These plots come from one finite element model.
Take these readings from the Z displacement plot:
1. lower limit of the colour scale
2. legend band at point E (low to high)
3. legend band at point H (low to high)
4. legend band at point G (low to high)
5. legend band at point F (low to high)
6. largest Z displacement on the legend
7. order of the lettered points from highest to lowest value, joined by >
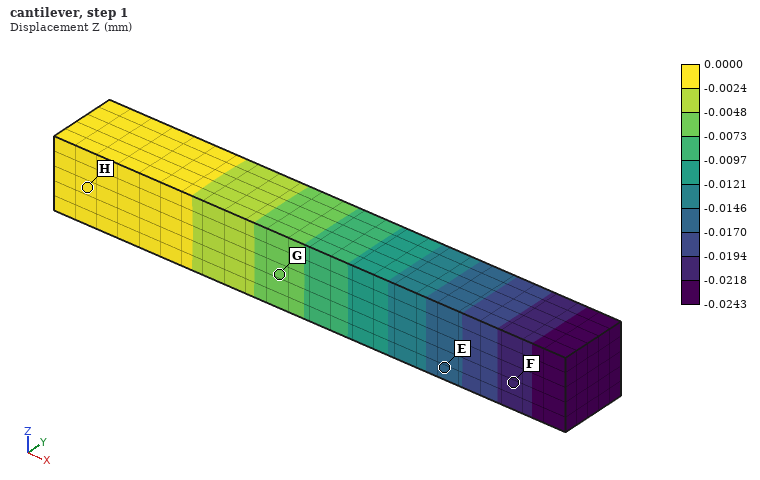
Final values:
-0.0243 mm
-0.0170 to -0.0146 mm
-0.0024 to 0.0000 mm
-0.0073 to -0.0048 mm
-0.0218 to -0.0194 mm
0.0000 mm
H > G > E > F
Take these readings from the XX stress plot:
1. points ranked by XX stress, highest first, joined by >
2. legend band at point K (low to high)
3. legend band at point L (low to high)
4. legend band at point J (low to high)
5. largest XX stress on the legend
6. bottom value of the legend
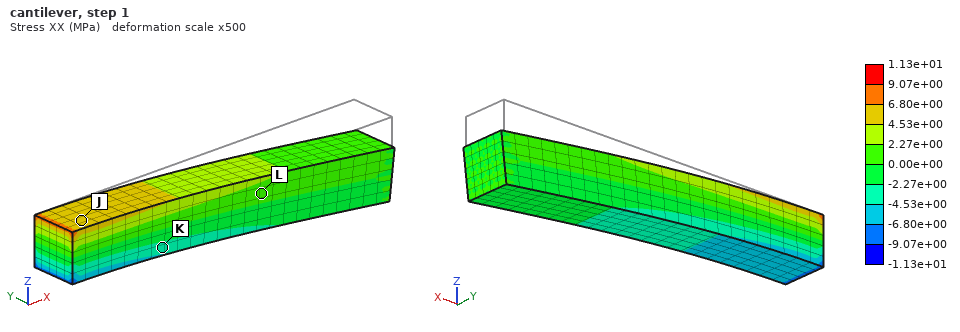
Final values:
J > L > K
-4.53e+00 to -2.27e+00 MPa
0.00e+00 to 2.27e+00 MPa
4.53e+00 to 6.80e+00 MPa
1.13e+01 MPa
-1.13e+01 MPa
